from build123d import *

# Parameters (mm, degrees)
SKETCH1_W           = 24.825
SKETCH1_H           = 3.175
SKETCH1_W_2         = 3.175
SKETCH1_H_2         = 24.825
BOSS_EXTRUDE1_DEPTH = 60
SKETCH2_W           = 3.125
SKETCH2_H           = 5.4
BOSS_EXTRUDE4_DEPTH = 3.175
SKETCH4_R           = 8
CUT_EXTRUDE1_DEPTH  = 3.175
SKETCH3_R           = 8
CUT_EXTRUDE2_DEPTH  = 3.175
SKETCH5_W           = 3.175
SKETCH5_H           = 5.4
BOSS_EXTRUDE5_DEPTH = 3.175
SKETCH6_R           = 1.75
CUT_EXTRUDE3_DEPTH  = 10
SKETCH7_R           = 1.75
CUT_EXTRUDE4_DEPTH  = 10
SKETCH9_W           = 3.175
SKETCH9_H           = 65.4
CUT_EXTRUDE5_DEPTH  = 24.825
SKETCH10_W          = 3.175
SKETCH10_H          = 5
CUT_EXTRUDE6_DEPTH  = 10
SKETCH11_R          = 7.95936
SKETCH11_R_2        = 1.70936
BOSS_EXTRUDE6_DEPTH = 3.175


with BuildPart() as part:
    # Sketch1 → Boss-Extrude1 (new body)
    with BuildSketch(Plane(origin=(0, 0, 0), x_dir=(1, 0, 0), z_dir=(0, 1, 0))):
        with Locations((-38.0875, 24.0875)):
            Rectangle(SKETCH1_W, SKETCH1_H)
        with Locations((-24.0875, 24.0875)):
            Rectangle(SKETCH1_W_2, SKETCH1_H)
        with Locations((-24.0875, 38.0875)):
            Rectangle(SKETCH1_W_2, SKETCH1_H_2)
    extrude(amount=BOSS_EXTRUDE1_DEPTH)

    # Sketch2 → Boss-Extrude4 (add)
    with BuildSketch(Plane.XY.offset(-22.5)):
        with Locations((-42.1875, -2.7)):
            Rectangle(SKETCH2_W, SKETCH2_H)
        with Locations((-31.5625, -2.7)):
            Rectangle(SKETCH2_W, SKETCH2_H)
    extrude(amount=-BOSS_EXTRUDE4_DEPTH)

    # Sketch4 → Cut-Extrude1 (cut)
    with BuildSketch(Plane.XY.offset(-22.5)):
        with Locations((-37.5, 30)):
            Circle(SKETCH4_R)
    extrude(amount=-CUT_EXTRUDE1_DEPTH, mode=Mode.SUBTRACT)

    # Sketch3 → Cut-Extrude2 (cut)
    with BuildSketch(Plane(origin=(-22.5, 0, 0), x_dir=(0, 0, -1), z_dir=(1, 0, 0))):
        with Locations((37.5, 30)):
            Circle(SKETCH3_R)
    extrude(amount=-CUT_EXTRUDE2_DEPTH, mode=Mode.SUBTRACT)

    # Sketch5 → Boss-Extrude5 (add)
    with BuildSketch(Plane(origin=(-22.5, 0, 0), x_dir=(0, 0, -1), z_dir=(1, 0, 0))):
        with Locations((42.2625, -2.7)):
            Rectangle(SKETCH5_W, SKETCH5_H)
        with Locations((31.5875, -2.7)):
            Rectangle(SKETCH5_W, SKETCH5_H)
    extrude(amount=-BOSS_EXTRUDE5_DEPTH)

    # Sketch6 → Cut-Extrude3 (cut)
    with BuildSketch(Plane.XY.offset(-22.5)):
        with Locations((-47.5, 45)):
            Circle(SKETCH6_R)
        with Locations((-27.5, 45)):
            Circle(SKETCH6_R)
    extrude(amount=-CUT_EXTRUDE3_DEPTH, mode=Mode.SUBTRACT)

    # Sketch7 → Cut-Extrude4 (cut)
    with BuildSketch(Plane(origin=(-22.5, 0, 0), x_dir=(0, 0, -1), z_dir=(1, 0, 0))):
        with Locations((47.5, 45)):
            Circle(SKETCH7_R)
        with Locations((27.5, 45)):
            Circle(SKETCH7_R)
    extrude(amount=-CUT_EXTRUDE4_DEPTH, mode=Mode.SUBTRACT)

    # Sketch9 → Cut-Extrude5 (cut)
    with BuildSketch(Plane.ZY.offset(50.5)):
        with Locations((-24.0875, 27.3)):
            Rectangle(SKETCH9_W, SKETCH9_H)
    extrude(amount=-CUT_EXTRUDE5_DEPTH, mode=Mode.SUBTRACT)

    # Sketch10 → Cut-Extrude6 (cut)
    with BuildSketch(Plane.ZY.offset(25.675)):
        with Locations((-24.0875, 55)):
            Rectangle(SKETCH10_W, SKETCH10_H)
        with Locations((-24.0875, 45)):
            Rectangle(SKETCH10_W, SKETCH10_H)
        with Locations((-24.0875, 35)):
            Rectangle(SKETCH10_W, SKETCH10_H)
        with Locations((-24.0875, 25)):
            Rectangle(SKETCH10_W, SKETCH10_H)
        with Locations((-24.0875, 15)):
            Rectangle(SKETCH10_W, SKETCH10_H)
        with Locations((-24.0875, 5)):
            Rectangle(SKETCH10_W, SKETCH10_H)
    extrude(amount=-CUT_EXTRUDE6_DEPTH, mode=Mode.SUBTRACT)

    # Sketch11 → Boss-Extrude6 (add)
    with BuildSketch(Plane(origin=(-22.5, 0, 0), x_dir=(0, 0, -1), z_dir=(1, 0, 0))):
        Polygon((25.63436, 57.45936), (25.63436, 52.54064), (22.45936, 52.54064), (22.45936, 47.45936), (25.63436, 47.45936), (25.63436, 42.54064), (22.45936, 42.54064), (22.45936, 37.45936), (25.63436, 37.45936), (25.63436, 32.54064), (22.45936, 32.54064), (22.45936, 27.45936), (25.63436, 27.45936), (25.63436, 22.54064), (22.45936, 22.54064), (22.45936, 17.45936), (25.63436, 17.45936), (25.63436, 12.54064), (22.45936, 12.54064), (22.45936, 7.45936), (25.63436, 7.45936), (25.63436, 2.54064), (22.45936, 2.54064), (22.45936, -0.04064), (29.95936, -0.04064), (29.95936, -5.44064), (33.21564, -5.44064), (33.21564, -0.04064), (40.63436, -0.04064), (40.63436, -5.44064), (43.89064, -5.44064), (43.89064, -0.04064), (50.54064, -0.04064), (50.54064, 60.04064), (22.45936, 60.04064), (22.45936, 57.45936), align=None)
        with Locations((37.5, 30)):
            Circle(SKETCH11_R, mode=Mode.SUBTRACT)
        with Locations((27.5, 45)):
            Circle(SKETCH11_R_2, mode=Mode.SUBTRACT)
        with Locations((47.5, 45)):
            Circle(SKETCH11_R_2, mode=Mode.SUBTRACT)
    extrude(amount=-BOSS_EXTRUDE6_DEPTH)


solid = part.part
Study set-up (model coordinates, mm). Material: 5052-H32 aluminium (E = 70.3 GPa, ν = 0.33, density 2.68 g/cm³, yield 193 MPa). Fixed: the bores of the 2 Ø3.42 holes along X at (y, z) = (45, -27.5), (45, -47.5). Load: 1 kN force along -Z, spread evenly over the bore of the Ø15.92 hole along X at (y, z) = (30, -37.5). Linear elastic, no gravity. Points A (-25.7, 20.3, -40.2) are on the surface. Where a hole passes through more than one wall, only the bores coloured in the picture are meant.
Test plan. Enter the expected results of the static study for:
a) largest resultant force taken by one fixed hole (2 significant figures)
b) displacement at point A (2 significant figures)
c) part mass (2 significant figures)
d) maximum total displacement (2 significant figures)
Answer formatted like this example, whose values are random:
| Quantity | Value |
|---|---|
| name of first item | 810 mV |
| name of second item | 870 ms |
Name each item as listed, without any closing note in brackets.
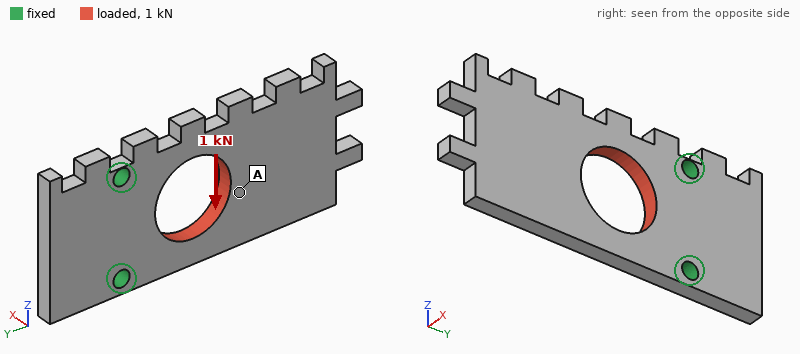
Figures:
| Quantity | Value |
|---|---|
| largest resultant force taken by one fixed hole | 850 N |
| displacement at point A | 49 µm |
| part mass | 12 g |
| maximum total displacement | 63 µm |
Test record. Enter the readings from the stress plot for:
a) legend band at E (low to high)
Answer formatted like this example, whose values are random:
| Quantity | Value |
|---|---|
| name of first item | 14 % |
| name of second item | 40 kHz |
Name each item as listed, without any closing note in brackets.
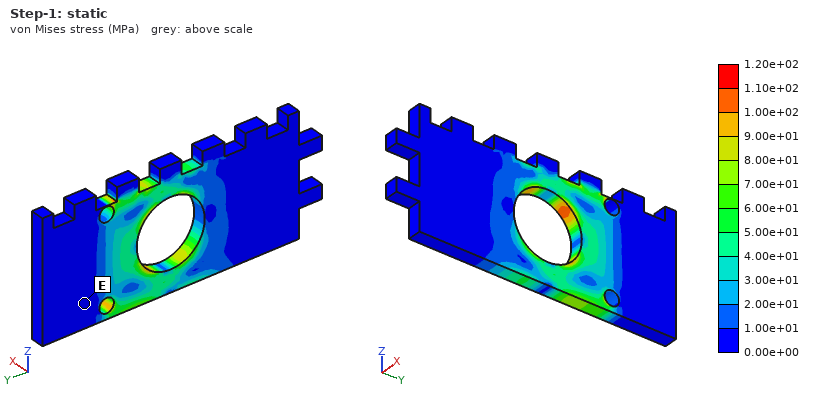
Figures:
| Quantity | Value |
|---|---|
| legend band at E | 0.00e+00 to 1.00e+01 MPa |
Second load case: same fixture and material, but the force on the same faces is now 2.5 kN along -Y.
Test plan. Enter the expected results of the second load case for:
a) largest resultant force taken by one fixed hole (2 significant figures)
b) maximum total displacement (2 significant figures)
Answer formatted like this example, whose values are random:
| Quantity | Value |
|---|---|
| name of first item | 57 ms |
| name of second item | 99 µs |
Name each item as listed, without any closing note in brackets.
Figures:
| Quantity | Value |
|---|---|
| largest resultant force taken by one fixed hole | 1.3 kN |
| maximum total displacement | 18 µm |
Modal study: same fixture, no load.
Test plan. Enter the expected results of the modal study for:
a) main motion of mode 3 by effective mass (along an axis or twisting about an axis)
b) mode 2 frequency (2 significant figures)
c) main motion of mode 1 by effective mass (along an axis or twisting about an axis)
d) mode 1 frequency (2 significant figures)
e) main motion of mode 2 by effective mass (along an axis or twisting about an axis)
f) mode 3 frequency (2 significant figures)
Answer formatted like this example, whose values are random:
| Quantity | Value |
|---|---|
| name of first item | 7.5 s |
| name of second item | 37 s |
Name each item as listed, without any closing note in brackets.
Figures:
| Quantity | Value |
|---|---|
| main motion of mode 3 by effective mass | along Z |
| mode 2 frequency | 3700 Hz |
| main motion of mode 1 by effective mass | along X |
| mode 1 frequency | 920 Hz |
| main motion of mode 2 by effective mass | twisting about Y |
| mode 3 frequency | 5600 Hz |
